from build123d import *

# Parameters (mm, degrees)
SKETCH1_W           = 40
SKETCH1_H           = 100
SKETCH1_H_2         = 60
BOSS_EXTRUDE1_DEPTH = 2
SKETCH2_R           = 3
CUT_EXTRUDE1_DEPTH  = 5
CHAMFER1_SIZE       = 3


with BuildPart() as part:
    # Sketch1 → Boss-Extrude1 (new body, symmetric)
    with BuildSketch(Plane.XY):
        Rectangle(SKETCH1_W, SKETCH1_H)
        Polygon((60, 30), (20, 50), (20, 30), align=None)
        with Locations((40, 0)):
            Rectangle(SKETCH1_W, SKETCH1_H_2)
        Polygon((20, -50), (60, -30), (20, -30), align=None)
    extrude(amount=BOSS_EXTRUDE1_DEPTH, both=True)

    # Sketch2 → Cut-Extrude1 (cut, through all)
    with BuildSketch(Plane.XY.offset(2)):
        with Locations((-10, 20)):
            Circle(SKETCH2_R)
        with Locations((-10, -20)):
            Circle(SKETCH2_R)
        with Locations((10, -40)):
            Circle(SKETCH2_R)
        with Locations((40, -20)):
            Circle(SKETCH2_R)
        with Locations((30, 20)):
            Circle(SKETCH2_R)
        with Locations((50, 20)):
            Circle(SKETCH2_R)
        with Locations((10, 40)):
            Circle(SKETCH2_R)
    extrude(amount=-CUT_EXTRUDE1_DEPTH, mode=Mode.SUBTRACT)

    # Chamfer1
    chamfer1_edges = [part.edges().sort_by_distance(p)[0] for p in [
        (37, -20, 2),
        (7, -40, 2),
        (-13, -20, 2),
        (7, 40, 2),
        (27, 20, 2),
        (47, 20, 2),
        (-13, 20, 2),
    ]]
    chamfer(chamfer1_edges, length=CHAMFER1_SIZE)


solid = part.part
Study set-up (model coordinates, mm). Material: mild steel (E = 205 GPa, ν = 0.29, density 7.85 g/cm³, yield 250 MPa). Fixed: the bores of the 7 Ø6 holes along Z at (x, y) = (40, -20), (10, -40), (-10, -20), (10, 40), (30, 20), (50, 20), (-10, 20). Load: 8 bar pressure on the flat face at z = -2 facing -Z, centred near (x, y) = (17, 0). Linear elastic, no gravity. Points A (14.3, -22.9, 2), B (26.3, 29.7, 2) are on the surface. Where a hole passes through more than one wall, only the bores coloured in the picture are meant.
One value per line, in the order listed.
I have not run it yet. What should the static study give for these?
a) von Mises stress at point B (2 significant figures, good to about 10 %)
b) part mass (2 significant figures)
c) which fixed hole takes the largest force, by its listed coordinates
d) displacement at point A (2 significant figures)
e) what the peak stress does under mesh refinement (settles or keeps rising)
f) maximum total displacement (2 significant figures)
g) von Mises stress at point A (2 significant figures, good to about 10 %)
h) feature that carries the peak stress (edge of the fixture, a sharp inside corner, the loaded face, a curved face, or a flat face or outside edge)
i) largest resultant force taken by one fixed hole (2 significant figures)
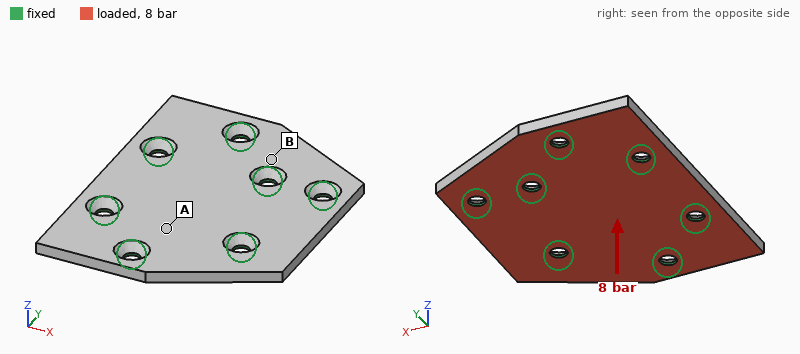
25 MPa
210 g
(40, -20)
7.8 µm
keeps rising
32 µm
13 MPa
edge of the fixture
1.2 kN
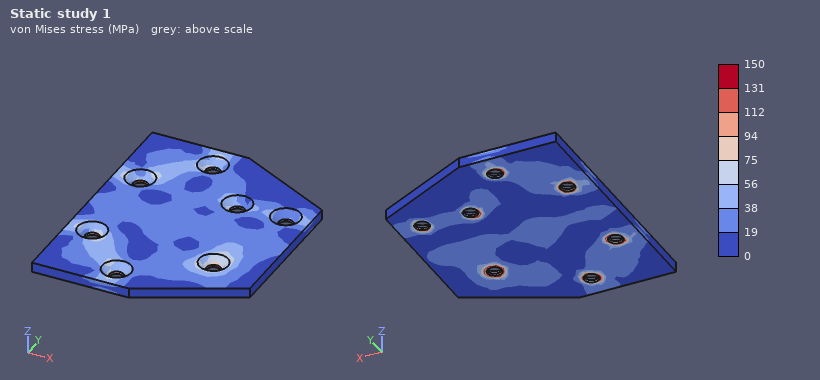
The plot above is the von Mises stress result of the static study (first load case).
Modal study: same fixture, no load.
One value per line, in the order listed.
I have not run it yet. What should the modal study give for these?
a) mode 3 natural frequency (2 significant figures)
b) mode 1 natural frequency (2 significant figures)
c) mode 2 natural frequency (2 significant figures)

6700 Hz
5500 Hz
5700 Hz
